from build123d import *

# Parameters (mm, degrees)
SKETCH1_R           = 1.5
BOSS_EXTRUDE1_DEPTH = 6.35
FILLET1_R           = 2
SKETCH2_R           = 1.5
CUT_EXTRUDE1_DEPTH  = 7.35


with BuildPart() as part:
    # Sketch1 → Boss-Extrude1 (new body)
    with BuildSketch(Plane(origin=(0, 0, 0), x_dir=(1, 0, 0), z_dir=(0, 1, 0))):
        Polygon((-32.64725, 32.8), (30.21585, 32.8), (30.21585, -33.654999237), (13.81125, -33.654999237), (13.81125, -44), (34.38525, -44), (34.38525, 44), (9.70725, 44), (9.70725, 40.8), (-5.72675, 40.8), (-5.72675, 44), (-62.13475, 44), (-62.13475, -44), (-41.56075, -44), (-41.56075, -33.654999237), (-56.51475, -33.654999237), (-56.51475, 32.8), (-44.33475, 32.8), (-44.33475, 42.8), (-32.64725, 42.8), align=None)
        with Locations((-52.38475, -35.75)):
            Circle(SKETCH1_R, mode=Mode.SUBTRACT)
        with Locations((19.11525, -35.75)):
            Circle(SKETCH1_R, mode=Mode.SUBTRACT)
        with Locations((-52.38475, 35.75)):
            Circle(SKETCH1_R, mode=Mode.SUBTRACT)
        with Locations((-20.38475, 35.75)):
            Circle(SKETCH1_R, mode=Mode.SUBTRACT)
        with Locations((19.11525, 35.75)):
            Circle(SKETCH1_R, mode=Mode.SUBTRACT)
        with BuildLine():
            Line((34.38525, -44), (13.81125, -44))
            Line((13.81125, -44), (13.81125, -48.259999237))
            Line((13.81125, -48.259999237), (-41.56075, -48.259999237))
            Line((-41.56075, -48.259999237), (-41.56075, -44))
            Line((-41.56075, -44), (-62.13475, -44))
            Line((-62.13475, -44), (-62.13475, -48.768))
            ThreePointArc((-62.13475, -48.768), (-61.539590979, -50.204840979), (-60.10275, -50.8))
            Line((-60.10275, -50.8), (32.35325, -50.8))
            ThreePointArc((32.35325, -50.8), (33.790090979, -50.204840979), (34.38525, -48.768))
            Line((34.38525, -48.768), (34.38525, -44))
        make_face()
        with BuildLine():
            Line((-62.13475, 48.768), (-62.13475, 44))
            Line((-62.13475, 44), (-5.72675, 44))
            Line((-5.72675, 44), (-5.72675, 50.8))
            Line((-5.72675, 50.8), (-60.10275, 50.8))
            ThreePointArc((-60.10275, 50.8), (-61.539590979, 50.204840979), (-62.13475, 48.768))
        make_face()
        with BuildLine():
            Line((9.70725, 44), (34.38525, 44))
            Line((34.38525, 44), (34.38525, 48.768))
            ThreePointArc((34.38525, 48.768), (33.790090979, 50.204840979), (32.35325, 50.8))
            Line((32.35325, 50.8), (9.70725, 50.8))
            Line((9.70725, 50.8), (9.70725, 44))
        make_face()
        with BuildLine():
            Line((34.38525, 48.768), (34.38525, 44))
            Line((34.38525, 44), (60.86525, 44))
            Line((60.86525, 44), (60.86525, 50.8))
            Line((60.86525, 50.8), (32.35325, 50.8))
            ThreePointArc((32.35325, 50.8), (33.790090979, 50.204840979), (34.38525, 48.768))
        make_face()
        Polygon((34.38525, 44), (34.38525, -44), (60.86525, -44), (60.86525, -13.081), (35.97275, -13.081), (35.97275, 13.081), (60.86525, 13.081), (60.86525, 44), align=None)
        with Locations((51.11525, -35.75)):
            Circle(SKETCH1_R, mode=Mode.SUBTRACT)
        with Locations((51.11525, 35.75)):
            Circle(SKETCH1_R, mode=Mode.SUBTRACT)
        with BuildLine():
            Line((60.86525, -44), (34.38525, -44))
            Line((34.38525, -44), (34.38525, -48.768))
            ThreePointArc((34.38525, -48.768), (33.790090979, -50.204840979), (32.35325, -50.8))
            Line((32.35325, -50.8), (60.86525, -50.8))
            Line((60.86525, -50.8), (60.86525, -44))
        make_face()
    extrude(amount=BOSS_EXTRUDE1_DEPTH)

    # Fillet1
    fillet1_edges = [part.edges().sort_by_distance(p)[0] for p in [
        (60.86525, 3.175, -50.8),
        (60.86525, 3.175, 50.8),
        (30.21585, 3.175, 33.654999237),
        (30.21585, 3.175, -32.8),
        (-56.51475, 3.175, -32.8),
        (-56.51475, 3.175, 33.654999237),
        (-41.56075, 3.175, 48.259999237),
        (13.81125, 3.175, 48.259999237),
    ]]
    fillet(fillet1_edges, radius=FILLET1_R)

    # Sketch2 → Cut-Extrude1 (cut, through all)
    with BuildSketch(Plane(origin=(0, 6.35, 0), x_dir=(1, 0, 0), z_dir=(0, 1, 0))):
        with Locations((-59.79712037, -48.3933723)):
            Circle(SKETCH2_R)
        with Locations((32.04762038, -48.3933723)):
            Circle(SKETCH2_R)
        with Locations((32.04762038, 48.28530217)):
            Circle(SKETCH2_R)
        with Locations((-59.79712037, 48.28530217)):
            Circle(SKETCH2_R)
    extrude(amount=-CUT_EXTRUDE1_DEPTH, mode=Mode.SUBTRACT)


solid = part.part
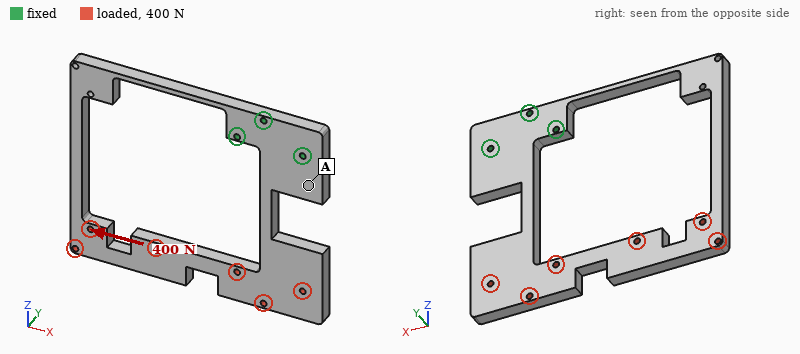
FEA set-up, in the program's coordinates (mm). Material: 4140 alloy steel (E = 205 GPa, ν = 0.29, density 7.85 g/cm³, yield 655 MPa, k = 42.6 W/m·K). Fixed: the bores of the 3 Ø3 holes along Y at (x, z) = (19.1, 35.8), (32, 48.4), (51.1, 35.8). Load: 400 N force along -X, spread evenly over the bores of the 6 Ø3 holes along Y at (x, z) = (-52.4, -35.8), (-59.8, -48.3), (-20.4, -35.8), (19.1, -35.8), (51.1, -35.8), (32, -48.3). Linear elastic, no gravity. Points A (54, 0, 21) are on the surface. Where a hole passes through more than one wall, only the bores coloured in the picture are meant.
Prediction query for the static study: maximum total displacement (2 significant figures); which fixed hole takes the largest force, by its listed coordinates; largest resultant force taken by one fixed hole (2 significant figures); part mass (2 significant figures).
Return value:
1.3 mm
(51.1, 35.8)
1.2 kN
250 g
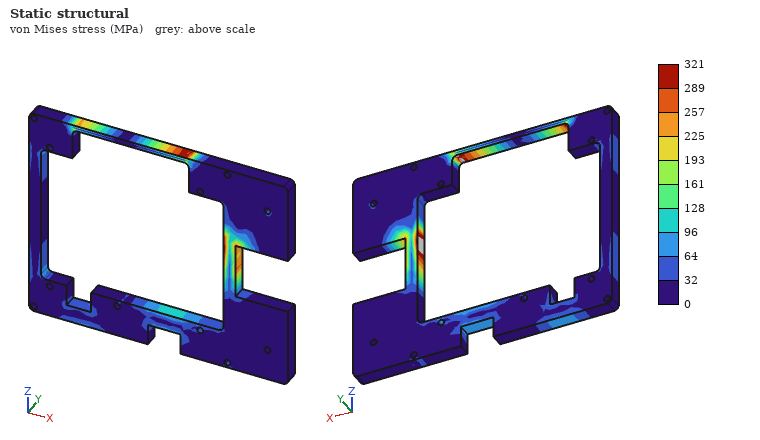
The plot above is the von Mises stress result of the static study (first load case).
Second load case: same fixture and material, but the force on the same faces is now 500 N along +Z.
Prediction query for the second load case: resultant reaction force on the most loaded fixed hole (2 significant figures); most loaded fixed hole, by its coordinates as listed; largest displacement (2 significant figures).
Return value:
610 N
(32, 48.4)
1.4 mm
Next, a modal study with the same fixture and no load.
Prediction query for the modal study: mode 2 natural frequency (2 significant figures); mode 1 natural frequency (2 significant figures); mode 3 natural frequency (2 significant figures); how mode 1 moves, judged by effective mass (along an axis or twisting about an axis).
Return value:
220 Hz
170 Hz
350 Hz
along Y
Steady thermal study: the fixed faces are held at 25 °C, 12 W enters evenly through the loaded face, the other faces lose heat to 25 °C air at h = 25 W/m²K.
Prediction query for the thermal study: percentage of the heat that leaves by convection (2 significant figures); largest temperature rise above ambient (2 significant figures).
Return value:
89 %
66 K
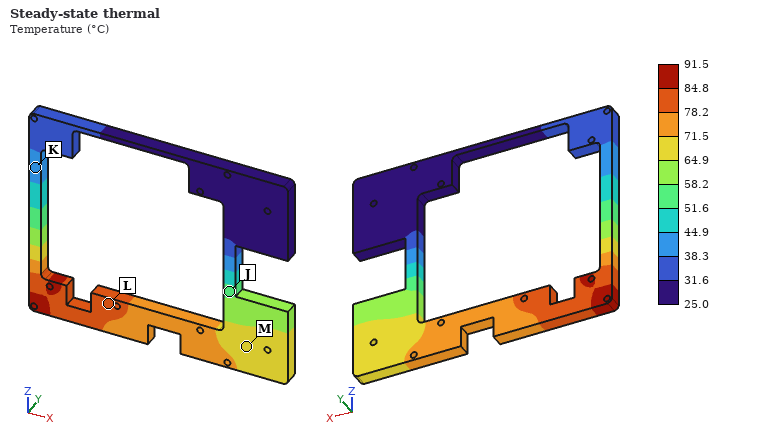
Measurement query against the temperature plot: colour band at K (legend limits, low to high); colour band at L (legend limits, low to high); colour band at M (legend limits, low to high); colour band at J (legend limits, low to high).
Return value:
38.3 to 44.9 °C
78.2 to 84.8 °C
64.9 to 71.5 °C
51.6 to 58.2 °C
